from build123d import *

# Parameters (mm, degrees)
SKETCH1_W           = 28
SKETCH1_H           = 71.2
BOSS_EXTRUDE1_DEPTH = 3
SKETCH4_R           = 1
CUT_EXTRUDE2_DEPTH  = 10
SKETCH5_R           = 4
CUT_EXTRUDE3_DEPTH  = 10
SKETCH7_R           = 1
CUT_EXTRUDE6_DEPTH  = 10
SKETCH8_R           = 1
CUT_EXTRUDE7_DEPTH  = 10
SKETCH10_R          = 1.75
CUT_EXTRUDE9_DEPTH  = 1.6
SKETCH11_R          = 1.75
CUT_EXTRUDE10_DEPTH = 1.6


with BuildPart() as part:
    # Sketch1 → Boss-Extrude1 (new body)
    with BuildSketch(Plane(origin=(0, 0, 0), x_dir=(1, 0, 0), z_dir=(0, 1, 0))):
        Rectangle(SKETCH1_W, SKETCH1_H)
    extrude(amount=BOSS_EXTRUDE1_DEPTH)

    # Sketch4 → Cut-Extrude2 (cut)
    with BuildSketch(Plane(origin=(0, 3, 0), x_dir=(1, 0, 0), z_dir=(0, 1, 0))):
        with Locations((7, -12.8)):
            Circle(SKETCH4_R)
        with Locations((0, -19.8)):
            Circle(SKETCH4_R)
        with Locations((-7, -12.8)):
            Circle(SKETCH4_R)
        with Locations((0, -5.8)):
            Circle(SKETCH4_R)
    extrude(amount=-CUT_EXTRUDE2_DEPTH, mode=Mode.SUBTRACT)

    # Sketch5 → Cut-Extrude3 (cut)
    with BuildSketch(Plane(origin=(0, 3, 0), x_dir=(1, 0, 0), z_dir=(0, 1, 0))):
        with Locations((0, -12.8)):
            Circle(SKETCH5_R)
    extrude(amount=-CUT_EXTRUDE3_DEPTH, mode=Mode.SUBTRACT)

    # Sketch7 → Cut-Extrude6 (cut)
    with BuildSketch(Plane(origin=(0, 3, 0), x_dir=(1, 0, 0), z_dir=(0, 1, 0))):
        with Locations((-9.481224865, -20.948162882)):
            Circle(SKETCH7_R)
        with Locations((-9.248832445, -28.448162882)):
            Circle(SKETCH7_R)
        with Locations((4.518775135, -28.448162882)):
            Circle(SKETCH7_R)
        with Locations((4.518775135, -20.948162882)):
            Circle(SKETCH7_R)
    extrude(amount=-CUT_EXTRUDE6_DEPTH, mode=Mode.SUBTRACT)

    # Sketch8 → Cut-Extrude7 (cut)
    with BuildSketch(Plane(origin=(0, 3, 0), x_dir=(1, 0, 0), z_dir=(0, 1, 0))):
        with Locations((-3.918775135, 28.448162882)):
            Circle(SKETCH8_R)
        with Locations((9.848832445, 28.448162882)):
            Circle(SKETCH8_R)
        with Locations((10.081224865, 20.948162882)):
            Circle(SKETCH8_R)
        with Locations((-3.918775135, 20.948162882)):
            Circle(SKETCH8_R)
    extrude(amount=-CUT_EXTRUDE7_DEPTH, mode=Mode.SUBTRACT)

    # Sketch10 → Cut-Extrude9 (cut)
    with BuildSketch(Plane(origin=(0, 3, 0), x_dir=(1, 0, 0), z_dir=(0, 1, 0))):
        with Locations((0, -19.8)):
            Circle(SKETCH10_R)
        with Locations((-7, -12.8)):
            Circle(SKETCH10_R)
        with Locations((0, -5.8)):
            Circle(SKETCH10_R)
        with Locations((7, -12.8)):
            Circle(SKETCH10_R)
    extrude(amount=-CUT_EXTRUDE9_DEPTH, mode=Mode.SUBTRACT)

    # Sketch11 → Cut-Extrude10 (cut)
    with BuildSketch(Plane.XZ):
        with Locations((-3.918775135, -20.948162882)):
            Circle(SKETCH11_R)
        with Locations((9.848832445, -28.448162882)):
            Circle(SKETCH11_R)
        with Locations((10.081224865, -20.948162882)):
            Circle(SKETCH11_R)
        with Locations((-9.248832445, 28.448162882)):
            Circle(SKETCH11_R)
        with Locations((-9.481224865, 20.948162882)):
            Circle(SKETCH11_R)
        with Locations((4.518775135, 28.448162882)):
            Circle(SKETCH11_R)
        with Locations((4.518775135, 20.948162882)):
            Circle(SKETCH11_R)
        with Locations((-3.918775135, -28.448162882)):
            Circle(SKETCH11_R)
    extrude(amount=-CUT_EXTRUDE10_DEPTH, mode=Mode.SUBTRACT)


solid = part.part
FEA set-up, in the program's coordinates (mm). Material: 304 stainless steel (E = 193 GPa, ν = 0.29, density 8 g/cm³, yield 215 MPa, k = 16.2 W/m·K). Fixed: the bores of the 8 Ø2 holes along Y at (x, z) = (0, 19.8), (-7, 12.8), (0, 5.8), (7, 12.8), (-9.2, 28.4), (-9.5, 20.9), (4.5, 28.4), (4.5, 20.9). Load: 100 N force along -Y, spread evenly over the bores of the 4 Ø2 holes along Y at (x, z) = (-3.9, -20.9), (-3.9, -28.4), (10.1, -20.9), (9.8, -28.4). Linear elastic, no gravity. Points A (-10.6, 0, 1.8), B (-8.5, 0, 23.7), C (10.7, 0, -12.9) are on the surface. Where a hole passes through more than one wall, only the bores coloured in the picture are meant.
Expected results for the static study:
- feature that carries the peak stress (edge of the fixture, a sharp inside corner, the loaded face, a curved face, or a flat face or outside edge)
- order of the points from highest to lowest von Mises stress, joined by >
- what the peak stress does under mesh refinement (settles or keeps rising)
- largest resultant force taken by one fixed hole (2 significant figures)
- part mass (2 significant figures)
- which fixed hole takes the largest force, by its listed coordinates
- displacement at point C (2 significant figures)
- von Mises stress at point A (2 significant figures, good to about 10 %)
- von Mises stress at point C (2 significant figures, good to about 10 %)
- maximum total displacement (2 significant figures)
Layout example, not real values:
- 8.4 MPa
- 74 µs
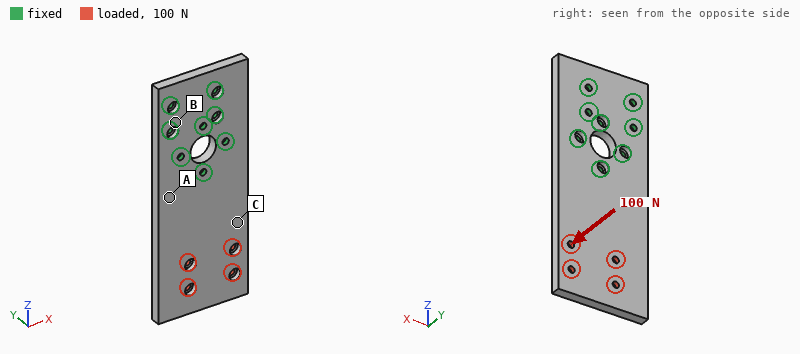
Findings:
- edge of the fixture
- A > C > B
- keeps rising
- 490 N
- 45 g
- (0, 5.8)
- 0.057 mm
- 54 MPa
- 28 MPa
- 0.16 mm
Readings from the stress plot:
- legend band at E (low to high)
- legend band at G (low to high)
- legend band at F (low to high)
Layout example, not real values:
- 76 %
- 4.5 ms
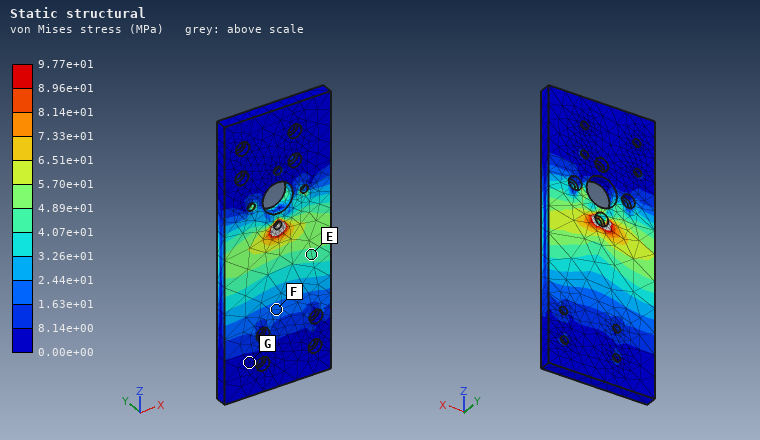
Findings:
- 4.07e+01 to 4.89e+01 MPa
- 0.00e+00 to 8.14e+00 MPa
- 1.63e+01 to 2.44e+01 MPa
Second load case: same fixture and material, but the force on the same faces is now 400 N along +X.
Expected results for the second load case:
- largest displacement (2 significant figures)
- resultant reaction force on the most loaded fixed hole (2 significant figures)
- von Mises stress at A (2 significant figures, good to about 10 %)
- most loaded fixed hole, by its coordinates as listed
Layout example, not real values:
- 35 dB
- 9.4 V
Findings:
- 19 µm
- 510 N
- 22 MPa
- (0, 5.8)
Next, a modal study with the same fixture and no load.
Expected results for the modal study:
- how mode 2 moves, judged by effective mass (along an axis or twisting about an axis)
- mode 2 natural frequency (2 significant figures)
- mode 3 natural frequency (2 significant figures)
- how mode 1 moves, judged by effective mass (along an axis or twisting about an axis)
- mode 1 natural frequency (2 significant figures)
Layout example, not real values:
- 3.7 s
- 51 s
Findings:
- twisting about Z
- 3500 Hz
- 6800 Hz
- along Y
- 1200 Hz
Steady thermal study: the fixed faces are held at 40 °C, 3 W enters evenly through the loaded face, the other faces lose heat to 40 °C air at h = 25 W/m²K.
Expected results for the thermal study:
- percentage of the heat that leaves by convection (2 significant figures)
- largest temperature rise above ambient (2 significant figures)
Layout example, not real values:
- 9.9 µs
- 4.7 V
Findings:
- 60 %
- 48 K
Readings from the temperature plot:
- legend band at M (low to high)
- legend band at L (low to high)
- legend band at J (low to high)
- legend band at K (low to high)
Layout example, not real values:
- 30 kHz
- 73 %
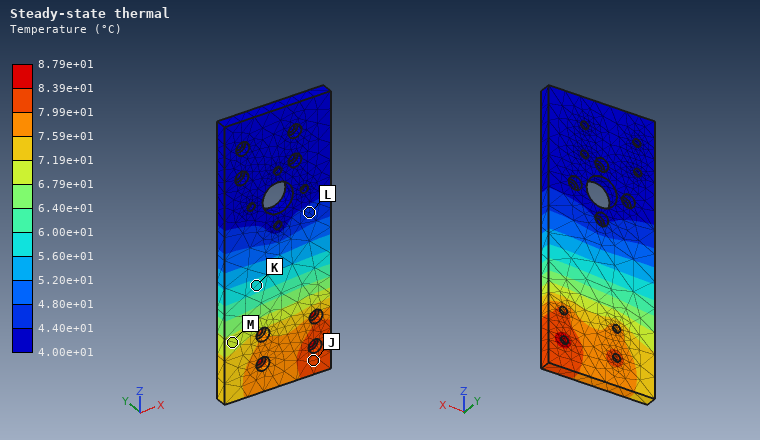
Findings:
- 6.79e+01 to 7.19e+01 °C
- 4.40e+01 to 4.80e+01 °C
- 7.99e+01 to 8.39e+01 °C
- 5.60e+01 to 6.00e+01 °C
